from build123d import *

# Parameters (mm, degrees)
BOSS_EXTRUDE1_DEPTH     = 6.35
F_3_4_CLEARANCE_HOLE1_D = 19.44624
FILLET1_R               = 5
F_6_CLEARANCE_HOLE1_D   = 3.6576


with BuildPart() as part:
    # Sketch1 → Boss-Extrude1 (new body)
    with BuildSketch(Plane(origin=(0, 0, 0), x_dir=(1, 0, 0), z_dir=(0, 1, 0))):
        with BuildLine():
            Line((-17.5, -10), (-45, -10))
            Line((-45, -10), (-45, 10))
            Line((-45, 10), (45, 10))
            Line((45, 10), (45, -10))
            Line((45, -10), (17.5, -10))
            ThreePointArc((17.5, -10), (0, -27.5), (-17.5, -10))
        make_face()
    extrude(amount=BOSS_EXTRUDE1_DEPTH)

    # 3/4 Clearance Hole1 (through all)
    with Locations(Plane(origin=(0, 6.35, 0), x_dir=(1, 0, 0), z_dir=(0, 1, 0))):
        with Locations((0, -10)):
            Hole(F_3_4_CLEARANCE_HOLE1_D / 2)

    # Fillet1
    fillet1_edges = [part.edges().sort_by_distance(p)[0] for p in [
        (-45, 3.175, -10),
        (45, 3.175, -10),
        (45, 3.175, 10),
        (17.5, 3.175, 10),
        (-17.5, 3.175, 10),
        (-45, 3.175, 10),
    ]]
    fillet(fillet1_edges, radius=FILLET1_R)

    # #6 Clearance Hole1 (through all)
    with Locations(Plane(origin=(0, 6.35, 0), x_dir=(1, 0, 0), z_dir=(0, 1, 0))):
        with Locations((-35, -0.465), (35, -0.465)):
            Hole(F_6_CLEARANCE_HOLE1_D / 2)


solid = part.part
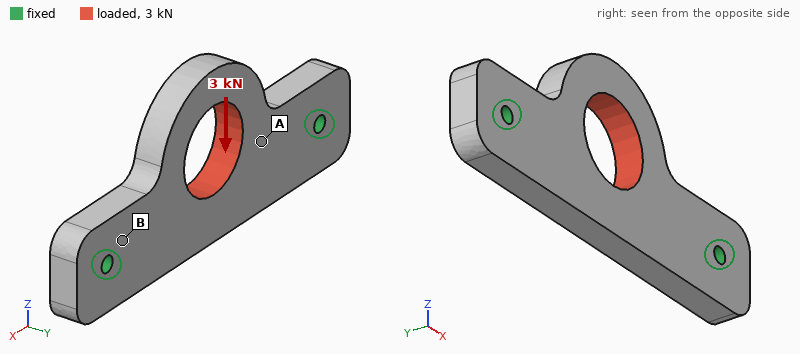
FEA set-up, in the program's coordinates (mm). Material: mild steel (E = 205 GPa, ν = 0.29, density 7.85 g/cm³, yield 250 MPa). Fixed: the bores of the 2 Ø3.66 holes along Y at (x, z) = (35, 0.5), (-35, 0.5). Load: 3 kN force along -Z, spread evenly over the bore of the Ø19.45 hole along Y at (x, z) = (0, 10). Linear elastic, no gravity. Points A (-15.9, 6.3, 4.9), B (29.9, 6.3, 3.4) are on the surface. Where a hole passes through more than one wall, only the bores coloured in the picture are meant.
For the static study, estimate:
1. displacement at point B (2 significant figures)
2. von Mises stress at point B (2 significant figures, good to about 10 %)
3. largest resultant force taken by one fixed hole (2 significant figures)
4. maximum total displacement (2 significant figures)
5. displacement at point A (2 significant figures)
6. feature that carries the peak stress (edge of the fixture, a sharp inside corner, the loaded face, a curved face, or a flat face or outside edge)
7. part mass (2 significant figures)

3.4 µm
30 MPa
1.6 kN
17 µm
12 µm
edge of the fixture
97 g
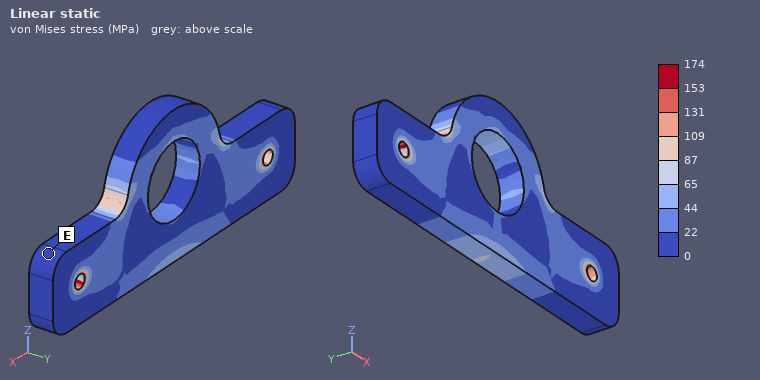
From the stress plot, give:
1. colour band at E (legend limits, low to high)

0 to 22 MPa
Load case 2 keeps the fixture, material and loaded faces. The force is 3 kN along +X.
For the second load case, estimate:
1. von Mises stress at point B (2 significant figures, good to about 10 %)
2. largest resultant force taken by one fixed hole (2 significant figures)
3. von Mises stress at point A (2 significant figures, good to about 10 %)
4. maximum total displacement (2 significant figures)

23 MPa
1.6 kN
8.4 MPa
6.2 µm
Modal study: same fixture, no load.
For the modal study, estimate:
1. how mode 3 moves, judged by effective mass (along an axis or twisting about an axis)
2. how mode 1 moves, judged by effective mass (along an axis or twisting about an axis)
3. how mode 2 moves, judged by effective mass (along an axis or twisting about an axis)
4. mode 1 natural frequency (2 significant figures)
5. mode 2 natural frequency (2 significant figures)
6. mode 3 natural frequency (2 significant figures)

along Z
along Y
along Y
4400 Hz
7100 Hz
10 kHz
